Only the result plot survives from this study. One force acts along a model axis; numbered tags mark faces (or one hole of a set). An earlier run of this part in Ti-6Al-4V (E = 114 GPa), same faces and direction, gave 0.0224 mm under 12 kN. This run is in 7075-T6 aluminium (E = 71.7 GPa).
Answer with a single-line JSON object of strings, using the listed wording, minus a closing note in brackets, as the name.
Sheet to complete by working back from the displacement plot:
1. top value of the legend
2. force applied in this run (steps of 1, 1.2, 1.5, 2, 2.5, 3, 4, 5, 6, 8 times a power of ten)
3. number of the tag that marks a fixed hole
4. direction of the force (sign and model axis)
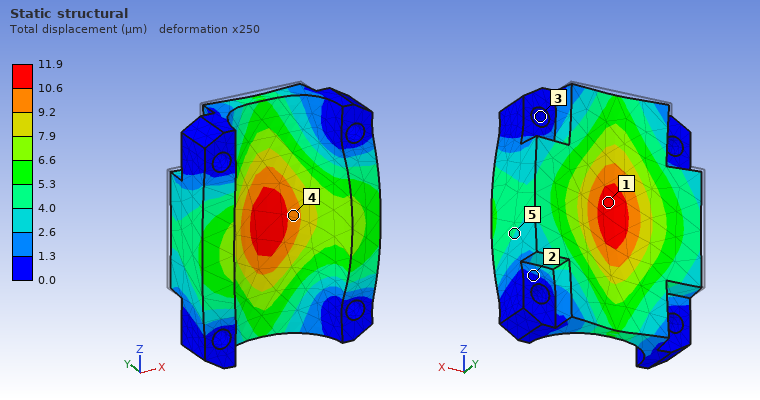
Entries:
{"top value of the legend": "11.9 µm", "force applied in this run": "4 kN", "number of the tag that marks a fixed hole": "3", "direction of the force": "-Y"}
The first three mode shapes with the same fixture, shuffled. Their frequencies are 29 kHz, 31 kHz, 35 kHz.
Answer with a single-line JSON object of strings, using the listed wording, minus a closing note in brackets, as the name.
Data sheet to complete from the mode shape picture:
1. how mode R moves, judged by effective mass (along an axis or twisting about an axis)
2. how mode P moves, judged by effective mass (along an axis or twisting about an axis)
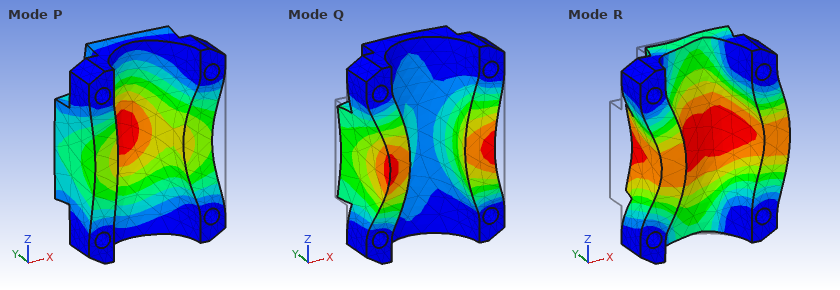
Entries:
{"how mode R moves, judged by effective mass": "along X", "how mode P moves, judged by effective mass": "along Y"}
